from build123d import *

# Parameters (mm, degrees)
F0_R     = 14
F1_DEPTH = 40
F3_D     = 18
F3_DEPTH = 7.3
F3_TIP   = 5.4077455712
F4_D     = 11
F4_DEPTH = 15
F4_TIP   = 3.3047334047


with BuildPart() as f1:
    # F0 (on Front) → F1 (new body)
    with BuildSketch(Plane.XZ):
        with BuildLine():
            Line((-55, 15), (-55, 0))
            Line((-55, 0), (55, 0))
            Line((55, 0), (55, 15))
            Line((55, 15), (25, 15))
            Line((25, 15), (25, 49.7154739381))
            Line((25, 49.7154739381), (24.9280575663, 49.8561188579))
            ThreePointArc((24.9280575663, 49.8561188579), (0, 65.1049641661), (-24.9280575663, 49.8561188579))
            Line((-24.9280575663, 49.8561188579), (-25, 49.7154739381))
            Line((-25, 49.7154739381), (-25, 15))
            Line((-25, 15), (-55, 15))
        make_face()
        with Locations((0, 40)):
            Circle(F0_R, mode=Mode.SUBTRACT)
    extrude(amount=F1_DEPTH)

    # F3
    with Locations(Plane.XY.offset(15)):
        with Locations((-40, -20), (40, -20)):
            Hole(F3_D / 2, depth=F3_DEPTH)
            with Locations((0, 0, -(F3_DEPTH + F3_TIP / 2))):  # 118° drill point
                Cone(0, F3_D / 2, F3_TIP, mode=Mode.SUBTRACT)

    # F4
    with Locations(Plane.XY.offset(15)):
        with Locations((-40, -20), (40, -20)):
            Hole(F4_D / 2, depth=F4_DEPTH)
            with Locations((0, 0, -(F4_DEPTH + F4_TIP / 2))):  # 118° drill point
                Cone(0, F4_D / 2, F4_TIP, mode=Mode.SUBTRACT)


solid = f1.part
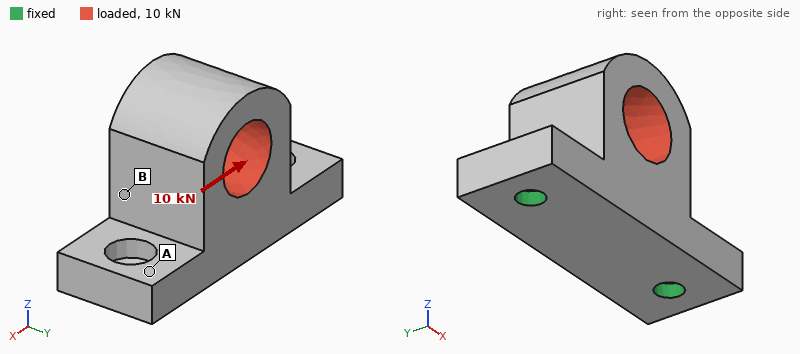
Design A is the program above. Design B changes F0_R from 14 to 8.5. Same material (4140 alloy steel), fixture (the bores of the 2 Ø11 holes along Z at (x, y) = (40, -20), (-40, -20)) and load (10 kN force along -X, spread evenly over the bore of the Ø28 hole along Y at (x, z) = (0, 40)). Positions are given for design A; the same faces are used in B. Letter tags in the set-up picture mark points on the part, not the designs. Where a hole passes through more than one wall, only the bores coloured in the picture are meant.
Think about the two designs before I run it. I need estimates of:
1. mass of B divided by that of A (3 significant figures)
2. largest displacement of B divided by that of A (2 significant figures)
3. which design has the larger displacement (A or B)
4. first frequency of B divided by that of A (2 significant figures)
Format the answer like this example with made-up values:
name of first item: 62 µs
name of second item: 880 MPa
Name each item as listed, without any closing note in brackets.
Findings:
mass of B divided by that of A: 1.12
largest displacement of B divided by that of A: 0.76
which design has the larger displacement: A
first frequency of B divided by that of A: 0.91
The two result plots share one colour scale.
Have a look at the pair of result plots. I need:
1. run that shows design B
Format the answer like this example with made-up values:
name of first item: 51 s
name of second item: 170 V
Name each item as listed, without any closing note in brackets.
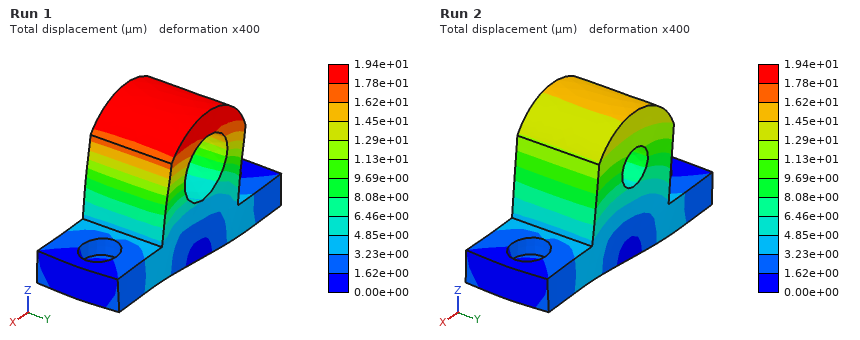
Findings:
run that shows design B: Run 2
